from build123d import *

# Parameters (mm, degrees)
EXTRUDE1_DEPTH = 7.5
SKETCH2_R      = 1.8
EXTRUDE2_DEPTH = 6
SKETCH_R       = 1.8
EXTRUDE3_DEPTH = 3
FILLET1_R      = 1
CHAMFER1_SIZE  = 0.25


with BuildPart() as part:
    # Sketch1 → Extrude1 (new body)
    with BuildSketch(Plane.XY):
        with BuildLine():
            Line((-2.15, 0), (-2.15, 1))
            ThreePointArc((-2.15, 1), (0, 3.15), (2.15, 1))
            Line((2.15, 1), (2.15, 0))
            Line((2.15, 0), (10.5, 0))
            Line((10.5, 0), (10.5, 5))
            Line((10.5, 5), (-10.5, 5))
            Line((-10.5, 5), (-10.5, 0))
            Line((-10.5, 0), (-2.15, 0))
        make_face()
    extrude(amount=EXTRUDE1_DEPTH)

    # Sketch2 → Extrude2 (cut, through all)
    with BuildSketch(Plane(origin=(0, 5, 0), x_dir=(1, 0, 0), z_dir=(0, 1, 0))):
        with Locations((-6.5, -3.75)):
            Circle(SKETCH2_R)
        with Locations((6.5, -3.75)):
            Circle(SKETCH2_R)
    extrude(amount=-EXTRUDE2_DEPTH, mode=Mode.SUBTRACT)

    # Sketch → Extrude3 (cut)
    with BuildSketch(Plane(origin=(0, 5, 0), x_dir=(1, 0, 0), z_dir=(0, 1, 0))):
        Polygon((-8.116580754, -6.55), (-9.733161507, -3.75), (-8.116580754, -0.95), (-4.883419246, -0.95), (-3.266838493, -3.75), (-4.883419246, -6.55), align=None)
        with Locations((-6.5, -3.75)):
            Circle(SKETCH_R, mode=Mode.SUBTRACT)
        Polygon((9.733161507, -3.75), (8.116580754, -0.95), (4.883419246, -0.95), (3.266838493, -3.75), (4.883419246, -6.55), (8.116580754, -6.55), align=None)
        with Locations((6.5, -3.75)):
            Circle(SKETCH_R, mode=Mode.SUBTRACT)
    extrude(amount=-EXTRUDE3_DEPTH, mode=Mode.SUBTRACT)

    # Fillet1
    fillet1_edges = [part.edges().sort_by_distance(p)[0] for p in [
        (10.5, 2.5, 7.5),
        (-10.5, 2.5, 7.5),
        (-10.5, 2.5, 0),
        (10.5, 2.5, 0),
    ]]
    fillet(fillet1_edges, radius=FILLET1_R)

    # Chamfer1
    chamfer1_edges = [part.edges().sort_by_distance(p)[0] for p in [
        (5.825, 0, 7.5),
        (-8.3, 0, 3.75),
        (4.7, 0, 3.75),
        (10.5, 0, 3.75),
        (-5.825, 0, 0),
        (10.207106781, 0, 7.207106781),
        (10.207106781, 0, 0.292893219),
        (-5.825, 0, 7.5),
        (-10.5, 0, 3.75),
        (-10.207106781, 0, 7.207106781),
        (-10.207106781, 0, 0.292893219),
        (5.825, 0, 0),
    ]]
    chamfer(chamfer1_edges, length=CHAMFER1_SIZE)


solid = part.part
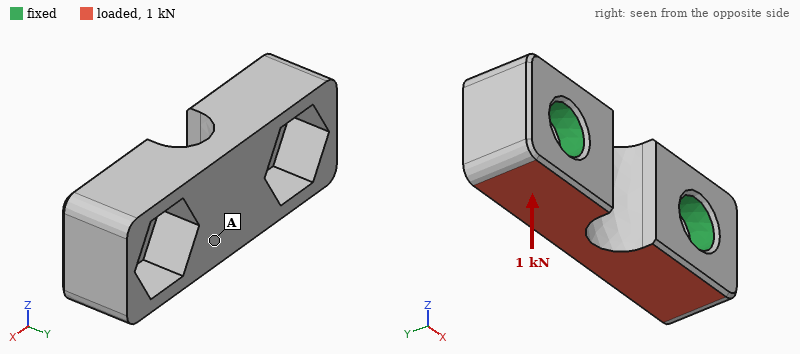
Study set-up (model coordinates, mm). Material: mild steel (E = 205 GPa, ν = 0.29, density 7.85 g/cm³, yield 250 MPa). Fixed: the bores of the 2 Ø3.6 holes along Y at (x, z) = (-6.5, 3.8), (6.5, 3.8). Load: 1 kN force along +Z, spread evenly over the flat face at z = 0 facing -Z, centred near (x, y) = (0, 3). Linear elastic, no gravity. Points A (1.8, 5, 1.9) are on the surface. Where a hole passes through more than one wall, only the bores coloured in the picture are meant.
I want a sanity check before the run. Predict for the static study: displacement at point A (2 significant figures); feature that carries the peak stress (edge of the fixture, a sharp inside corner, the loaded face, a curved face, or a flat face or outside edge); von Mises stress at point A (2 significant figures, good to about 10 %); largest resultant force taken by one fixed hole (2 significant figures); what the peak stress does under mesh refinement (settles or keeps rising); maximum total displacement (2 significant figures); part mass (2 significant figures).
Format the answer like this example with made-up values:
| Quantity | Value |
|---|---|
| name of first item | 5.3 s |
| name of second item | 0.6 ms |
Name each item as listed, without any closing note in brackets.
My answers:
| Quantity | Value |
|---|---|
| displacement at point A | 2.8 µm |
| feature that carries the peak stress | edge of the fixture |
| von Mises stress at point A | 20 MPa |
| largest resultant force taken by one fixed hole | 500 N |
| what the peak stress does under mesh refinement | keeps rising |
| maximum total displacement | 4.3 µm |
| part mass | 3.9 g |
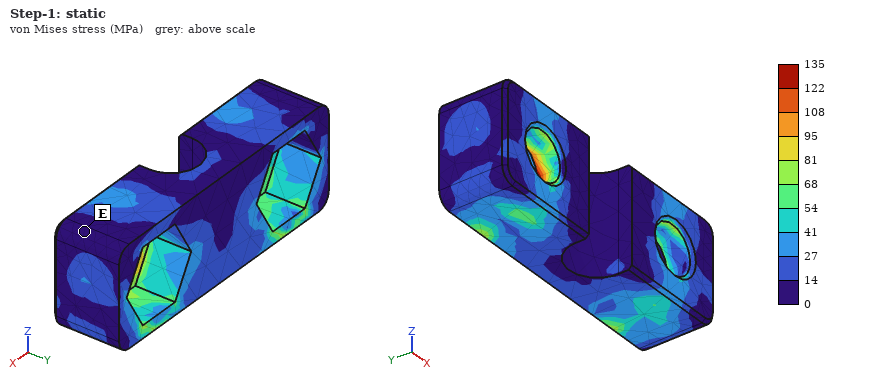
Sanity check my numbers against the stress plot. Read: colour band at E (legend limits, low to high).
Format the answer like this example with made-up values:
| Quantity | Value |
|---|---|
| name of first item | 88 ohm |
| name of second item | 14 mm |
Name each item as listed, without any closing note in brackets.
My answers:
| Quantity | Value |
|---|---|
| colour band at E | 0 to 14 MPa |
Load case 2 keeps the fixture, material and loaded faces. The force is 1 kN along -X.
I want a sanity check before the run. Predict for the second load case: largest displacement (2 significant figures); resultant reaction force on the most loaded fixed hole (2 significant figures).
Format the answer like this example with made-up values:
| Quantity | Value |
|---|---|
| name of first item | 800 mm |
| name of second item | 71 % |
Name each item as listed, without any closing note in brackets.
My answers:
| Quantity | Value |
|---|---|
| largest displacement | 2.6 µm |
| resultant reaction force on the most loaded fixed hole | 530 N |
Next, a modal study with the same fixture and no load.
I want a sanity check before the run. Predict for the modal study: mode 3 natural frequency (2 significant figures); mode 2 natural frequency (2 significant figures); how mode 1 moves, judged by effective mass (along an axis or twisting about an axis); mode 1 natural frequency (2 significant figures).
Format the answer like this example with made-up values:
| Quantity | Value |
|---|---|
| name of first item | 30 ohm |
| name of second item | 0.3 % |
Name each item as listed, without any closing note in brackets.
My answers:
| Quantity | Value |
|---|---|
| mode 3 natural frequency | 79 kHz |
| mode 2 natural frequency | 77 kHz |
| how mode 1 moves, judged by effective mass | along Z |
| mode 1 natural frequency | 55 kHz |
